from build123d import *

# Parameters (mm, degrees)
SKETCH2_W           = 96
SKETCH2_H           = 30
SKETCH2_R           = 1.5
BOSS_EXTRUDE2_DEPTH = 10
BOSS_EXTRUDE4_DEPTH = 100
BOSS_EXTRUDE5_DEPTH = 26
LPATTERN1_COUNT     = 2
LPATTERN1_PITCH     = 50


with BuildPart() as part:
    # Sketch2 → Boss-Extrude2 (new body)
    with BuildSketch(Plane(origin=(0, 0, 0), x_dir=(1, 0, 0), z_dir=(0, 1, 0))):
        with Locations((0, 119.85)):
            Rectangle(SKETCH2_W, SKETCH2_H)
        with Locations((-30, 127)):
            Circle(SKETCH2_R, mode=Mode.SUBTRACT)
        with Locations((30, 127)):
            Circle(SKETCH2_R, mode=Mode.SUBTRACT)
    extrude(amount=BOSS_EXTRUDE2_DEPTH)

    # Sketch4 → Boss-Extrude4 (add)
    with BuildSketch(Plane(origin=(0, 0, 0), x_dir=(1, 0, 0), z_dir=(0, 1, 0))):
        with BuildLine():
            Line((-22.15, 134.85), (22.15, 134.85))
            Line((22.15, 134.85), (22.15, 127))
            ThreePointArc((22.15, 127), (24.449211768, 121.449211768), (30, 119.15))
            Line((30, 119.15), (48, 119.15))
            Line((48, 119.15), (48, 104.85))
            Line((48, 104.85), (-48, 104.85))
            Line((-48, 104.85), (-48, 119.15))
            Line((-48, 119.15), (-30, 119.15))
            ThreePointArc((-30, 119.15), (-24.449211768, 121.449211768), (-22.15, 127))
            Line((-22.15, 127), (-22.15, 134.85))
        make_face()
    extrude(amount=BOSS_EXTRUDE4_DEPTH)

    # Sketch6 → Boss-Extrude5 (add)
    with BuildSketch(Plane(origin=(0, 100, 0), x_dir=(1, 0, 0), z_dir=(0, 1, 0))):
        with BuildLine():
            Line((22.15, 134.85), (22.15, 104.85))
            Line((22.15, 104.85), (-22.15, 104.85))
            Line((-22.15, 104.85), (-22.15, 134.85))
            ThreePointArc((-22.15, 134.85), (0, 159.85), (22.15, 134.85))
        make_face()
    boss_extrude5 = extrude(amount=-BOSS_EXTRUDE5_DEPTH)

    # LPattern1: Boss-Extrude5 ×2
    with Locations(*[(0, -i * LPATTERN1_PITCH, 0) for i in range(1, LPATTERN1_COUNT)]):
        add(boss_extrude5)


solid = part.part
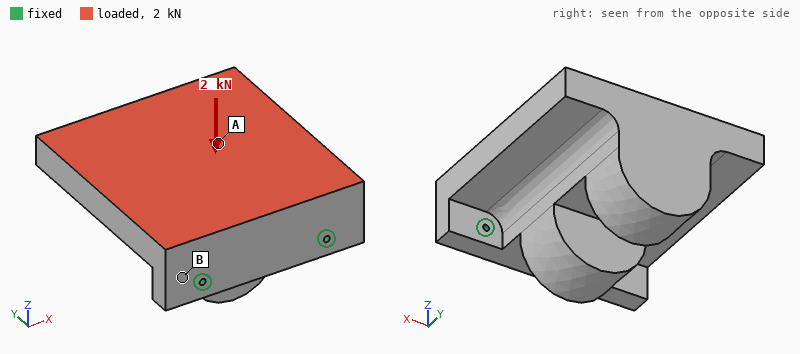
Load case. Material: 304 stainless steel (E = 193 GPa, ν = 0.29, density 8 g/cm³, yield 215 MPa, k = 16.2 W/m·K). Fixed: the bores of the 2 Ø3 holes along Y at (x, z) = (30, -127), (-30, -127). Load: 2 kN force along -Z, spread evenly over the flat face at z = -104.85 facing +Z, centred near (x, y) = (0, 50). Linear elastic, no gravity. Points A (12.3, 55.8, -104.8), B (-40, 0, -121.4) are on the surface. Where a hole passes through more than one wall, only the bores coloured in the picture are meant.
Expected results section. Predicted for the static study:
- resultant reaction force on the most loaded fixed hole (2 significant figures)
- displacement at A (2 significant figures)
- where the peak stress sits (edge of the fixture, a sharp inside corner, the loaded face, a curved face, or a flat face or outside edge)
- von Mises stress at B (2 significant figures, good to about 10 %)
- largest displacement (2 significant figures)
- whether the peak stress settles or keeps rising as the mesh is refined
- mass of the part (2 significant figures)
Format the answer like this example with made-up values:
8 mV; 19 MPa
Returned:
1.1 kN; 0.070 mm; edge of the fixture; 31 MPa; 0.13 mm; keeps rising; 2.1 kg
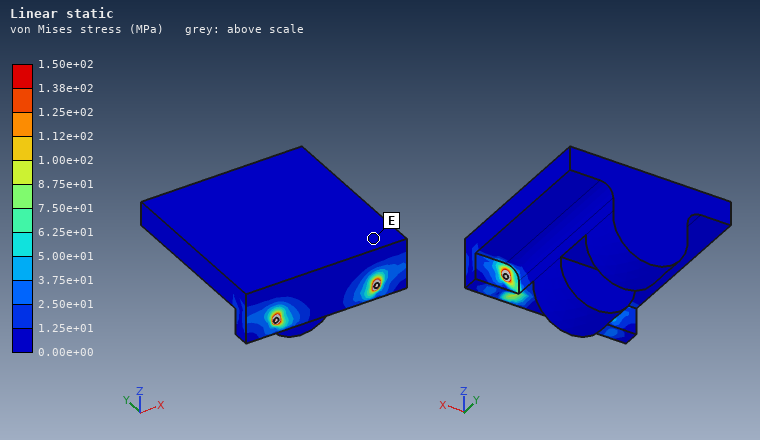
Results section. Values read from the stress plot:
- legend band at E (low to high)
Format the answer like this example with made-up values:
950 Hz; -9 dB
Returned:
0.00e+00 to 1.25e+01 MPa
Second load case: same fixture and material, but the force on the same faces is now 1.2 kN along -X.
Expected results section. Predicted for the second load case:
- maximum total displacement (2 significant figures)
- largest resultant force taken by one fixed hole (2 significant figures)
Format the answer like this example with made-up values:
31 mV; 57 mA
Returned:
4.9 µm; 1.2 kN
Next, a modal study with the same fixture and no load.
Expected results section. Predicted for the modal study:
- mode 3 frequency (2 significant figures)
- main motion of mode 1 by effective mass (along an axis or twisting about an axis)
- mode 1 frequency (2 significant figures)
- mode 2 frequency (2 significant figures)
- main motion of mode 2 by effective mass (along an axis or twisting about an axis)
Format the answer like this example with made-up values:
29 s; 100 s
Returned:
3700 Hz; along Z; 520 Hz; 2000 Hz; along X
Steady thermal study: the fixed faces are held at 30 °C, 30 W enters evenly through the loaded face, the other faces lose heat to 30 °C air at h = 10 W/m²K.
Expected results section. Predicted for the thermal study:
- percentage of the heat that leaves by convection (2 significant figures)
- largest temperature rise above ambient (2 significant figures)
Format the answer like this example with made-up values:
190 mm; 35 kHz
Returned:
35 %; 54 K
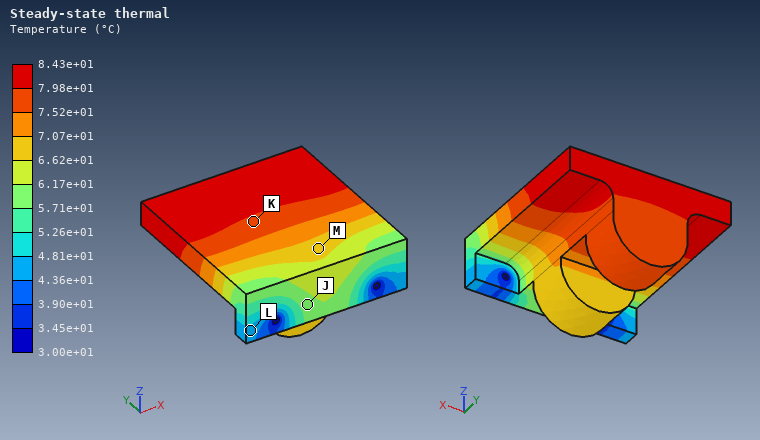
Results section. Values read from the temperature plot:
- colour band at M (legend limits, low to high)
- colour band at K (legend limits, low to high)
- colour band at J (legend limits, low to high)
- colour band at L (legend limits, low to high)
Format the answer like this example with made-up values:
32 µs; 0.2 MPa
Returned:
6.62e+01 to 7.07e+01 °C; 7.52e+01 to 7.98e+01 °C; 5.71e+01 to 6.17e+01 °C; 4.36e+01 to 4.81e+01 °C
